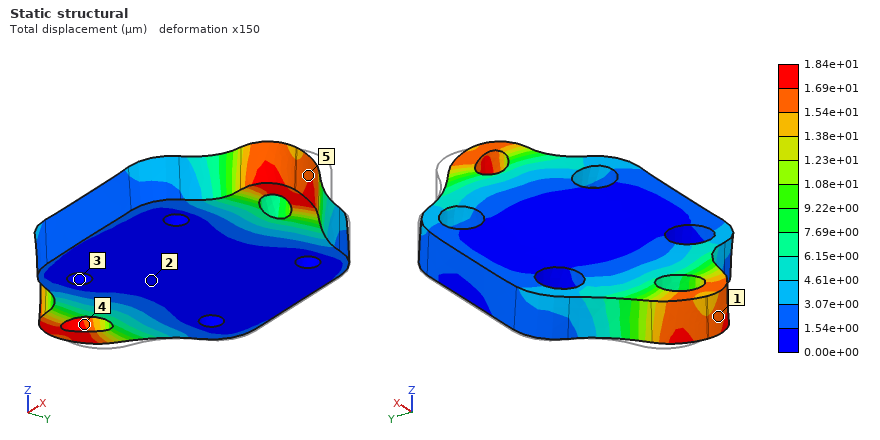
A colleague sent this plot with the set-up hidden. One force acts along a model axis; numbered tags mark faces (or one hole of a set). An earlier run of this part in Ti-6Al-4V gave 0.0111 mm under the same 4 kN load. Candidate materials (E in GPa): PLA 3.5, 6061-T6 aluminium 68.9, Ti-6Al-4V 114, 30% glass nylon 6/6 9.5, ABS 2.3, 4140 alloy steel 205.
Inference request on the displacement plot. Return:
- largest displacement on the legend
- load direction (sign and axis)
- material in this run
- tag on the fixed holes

1.84e+01 µm
-Y
6061-T6 aluminium
3
